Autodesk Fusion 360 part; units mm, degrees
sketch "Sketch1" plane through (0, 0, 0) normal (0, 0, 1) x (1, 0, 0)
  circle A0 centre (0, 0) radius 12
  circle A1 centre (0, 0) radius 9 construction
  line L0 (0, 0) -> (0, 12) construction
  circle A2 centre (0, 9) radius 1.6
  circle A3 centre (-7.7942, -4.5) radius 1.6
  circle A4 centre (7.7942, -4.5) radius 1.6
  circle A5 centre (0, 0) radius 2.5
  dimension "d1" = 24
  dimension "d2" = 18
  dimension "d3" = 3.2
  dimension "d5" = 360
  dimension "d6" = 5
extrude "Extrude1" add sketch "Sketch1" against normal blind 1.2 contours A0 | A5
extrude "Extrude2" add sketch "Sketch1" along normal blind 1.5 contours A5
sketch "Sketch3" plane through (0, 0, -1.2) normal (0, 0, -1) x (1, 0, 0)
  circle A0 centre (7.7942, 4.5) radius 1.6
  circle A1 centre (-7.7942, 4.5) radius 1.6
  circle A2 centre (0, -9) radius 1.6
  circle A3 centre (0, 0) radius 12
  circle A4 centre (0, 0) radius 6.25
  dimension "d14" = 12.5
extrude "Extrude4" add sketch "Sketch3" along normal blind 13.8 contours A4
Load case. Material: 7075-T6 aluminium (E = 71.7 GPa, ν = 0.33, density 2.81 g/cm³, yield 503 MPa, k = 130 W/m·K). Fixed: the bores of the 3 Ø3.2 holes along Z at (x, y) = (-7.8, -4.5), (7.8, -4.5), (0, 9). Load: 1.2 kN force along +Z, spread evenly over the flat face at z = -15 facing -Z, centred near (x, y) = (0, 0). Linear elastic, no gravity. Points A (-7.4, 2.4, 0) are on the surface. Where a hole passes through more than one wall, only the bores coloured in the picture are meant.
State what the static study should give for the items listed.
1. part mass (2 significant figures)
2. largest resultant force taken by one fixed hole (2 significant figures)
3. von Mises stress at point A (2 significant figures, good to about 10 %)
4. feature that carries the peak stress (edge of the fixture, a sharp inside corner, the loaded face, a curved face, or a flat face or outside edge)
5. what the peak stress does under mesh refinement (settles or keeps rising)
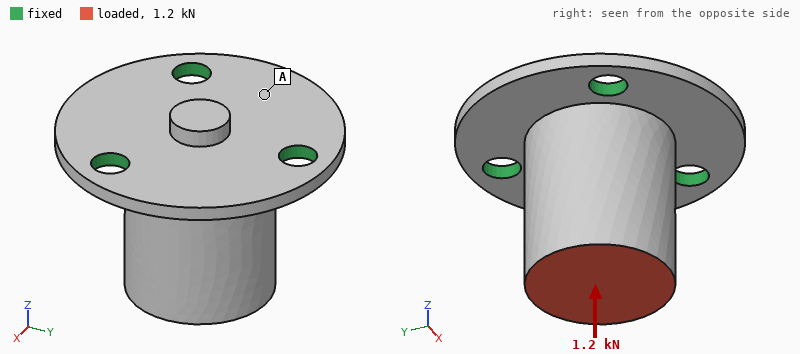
6.3 g
440 N
27 MPa
edge of the fixture
keeps rising
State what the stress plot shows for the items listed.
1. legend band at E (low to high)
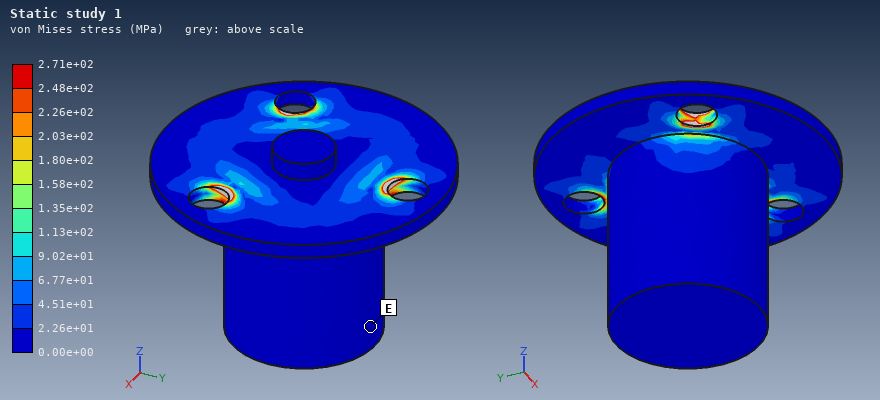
0.00e+00 to 2.26e+01 MPa
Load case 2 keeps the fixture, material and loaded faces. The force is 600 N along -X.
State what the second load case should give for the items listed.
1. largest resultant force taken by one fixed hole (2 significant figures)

740 N
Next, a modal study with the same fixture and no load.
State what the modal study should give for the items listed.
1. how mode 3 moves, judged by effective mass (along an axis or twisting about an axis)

along Z
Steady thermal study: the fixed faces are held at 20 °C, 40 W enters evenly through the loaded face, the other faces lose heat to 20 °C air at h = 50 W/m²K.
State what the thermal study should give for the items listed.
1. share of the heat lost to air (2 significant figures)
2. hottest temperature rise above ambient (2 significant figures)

4.6 %
62 K
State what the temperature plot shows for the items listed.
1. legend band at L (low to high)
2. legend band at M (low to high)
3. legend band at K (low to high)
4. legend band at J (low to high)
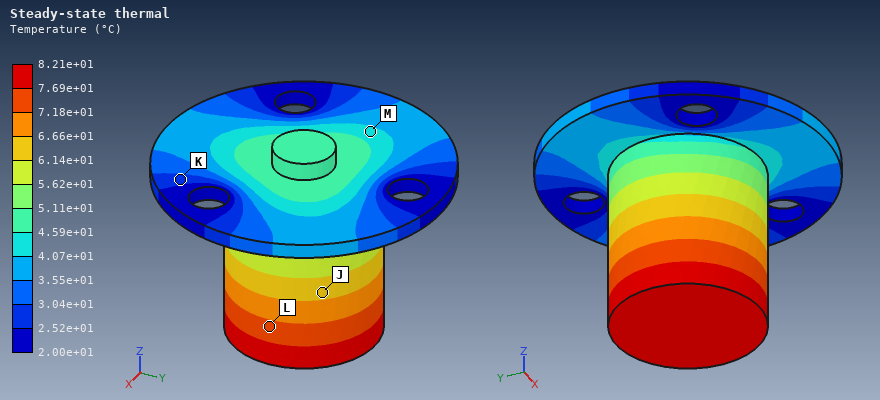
7.18e+01 to 7.69e+01 °C
4.07e+01 to 4.59e+01 °C
2.52e+01 to 3.04e+01 °C
6.14e+01 to 6.66e+01 °C
